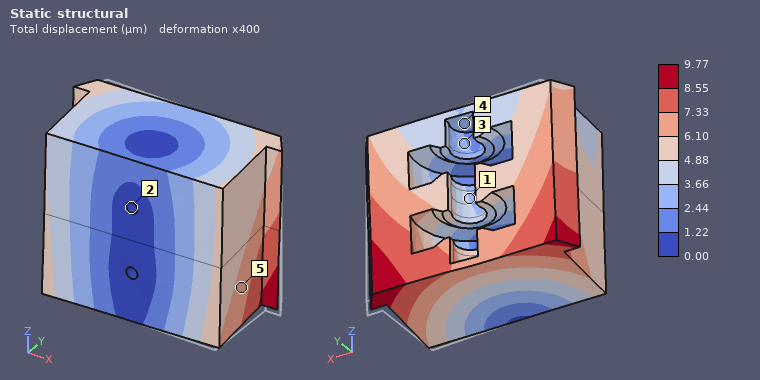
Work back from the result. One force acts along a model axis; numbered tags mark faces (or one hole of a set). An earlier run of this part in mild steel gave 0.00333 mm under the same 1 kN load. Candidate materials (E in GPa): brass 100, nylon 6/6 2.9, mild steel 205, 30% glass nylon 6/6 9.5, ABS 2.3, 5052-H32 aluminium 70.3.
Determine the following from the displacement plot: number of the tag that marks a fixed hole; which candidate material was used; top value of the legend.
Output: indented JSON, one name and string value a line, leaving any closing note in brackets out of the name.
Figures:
{
  "number of the tag that marks a fixed hole": "2",
  "which candidate material was used": "5052-H32 aluminium",
  "top value of the legend": "9.77 µm"
}
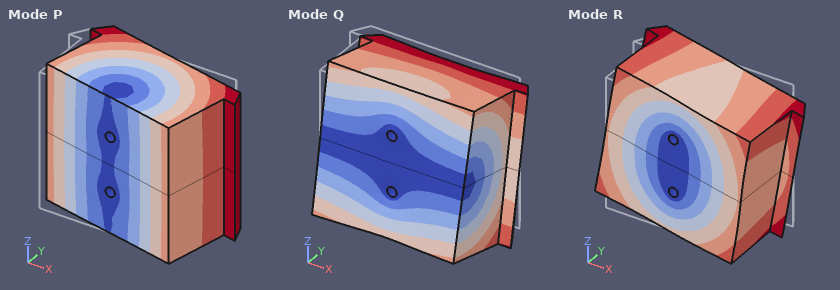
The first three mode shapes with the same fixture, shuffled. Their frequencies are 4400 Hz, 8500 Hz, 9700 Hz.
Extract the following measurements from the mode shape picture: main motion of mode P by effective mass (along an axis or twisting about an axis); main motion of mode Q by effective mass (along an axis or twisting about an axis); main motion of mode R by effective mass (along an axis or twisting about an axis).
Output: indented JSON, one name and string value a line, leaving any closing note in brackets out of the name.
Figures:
{
  "main motion of mode P by effective mass": "along X",
  "main motion of mode Q by effective mass": "along Z",
  "main motion of mode R by effective mass": "twisting about Y"
}
